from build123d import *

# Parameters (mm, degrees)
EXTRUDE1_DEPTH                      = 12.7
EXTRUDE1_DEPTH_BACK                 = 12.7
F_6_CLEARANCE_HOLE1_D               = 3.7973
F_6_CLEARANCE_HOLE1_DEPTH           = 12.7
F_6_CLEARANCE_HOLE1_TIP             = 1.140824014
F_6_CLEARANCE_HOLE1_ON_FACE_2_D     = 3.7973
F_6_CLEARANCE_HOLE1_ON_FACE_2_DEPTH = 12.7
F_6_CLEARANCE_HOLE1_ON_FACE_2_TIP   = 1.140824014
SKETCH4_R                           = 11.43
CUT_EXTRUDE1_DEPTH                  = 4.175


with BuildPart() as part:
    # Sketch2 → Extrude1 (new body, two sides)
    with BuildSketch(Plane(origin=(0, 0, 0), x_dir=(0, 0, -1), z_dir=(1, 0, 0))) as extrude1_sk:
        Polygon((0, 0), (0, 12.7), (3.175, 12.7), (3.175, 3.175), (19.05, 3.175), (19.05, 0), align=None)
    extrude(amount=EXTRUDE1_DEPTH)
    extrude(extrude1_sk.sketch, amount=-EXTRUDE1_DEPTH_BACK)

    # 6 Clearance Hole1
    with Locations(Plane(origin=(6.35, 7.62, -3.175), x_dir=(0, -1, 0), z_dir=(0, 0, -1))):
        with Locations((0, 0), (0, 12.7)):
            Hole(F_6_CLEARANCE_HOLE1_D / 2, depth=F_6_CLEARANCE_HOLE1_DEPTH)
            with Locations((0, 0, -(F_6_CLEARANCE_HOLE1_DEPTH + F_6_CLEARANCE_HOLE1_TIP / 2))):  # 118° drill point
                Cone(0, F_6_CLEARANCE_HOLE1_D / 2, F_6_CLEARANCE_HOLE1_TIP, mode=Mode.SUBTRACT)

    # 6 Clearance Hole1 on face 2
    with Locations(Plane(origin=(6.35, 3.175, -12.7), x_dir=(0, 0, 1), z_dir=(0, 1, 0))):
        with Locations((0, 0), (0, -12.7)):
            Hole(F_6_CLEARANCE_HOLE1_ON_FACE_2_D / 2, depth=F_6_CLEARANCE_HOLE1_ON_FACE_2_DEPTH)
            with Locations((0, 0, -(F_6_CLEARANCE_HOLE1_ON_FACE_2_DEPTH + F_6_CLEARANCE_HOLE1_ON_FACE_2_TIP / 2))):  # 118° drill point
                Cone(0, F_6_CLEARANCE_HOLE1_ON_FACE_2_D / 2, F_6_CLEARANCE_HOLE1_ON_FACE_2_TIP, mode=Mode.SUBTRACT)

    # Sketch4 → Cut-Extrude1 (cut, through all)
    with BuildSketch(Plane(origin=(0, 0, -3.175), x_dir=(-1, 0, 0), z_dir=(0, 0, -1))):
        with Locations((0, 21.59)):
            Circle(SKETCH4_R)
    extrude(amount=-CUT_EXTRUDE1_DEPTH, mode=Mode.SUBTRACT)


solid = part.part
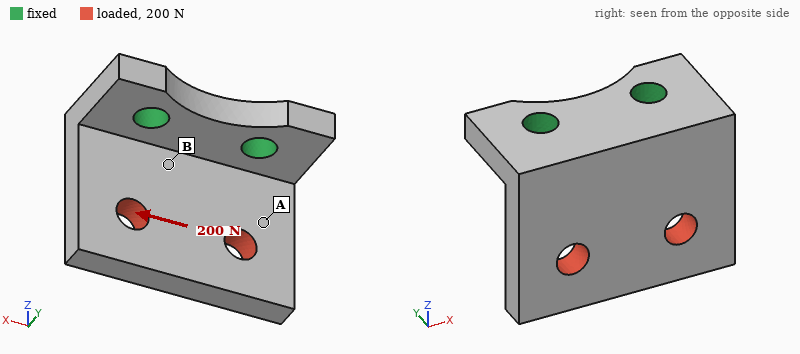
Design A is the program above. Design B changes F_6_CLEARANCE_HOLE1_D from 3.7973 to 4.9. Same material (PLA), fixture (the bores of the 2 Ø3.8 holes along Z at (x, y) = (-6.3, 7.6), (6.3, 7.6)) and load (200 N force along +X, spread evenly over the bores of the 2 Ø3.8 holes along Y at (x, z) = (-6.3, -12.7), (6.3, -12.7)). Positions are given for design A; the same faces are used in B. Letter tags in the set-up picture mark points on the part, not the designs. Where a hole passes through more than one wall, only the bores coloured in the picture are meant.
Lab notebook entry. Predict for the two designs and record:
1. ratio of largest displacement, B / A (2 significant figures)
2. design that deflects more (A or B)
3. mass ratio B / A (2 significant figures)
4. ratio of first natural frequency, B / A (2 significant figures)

0.81
A
0.98
1.1
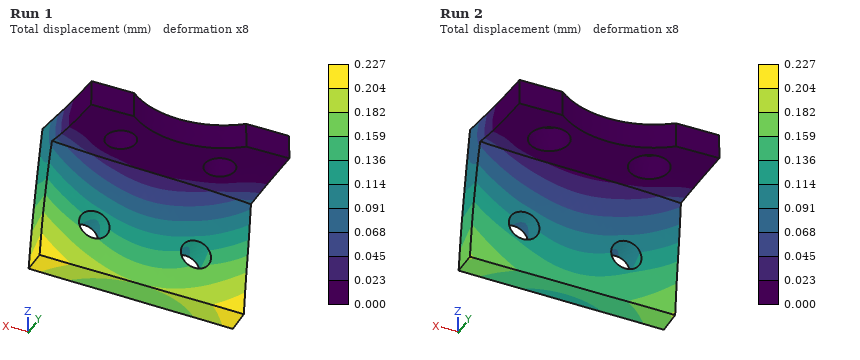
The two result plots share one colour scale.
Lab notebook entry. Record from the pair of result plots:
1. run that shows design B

Run 2
